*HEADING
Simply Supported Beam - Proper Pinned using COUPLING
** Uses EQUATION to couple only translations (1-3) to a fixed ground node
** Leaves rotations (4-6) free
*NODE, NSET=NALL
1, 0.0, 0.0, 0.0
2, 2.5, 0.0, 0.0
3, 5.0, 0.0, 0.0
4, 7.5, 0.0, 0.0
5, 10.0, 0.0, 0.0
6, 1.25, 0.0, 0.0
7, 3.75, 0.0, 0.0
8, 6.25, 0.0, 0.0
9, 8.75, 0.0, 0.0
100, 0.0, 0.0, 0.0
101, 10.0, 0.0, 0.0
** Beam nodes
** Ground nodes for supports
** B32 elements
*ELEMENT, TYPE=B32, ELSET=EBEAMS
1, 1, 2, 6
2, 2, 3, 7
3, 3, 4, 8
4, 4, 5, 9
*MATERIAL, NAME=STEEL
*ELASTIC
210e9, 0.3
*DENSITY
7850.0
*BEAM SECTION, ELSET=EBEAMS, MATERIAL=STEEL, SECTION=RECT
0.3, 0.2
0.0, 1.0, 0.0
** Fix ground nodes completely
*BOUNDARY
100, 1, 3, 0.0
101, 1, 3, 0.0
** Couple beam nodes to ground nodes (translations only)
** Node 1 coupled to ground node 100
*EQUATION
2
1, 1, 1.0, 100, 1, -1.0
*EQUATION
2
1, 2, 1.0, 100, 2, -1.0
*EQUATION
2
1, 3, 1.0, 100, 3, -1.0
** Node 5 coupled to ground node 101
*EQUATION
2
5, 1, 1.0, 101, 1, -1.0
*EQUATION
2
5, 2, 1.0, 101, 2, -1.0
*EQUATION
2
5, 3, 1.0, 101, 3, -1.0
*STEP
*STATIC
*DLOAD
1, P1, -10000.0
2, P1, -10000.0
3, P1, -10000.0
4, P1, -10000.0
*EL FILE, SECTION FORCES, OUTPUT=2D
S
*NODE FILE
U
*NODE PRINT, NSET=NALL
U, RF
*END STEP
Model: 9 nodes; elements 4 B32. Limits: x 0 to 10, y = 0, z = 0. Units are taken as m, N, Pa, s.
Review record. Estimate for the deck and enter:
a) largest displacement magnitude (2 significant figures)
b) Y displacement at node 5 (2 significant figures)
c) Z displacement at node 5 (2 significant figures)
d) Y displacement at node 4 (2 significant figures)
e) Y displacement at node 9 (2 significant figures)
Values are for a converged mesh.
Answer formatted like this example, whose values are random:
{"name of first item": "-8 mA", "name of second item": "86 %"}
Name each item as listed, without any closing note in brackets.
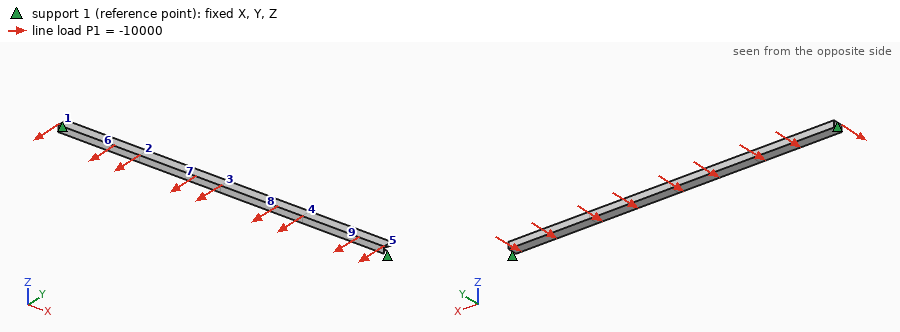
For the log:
{"largest displacement magnitude": "0.053 m", "Y displacement at node 5": "-0.021 m", "Z displacement at node 5": "-0.032 m", "Y displacement at node 4": "-0.036 m", "Y displacement at node 9": "0.013 m"}
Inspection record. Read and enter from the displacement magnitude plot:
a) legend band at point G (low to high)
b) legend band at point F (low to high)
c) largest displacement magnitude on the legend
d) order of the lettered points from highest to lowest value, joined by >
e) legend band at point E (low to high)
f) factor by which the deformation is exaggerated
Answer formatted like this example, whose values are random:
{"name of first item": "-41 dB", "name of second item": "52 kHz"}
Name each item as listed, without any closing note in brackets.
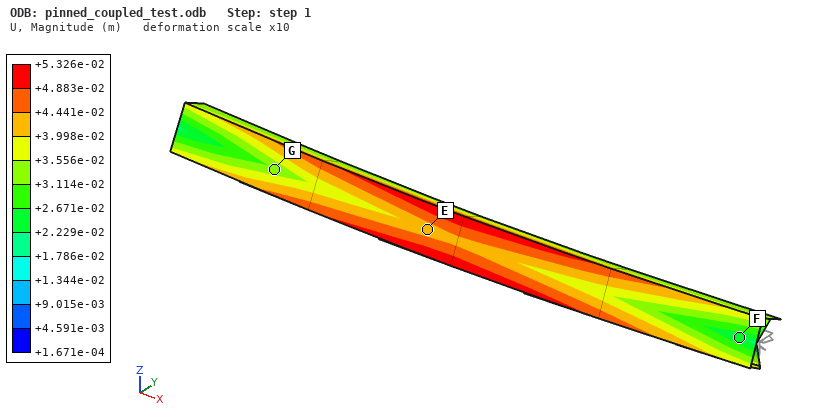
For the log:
{"legend band at point G": "+3.114e-02 to +3.556e-02 m", "legend band at point F": "+2.229e-02 to +2.671e-02 m", "largest displacement magnitude on the legend": "+5.326e-02 m", "order of the lettered points from highest to lowest value, joined by >": "E > G > F", "legend band at point E": "+3.998e-02 to +4.441e-02 m", "factor by which the deformation is exaggerated": "10"}
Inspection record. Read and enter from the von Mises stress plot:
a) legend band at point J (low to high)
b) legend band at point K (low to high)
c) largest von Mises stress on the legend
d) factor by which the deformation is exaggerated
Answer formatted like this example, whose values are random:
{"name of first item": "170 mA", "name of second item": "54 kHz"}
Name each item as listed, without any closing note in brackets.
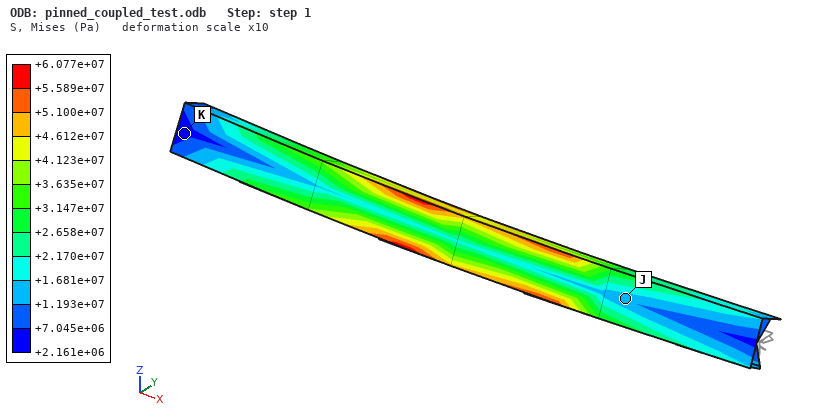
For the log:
{"legend band at point J": "+1.193e+07 to +1.681e+07 Pa", "legend band at point K": "+2.161e+06 to +7.045e+06 Pa", "largest von Mises stress on the legend": "+6.077e+07 Pa", "factor by which the deformation is exaggerated": "10"}
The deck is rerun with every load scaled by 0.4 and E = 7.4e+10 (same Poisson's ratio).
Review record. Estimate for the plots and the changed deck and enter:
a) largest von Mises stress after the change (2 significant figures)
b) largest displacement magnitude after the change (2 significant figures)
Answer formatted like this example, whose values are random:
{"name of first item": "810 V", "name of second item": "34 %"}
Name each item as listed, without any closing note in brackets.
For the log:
{"largest von Mises stress after the change": "2.4e+07 Pa", "largest displacement magnitude after the change": "0.060 m"}
